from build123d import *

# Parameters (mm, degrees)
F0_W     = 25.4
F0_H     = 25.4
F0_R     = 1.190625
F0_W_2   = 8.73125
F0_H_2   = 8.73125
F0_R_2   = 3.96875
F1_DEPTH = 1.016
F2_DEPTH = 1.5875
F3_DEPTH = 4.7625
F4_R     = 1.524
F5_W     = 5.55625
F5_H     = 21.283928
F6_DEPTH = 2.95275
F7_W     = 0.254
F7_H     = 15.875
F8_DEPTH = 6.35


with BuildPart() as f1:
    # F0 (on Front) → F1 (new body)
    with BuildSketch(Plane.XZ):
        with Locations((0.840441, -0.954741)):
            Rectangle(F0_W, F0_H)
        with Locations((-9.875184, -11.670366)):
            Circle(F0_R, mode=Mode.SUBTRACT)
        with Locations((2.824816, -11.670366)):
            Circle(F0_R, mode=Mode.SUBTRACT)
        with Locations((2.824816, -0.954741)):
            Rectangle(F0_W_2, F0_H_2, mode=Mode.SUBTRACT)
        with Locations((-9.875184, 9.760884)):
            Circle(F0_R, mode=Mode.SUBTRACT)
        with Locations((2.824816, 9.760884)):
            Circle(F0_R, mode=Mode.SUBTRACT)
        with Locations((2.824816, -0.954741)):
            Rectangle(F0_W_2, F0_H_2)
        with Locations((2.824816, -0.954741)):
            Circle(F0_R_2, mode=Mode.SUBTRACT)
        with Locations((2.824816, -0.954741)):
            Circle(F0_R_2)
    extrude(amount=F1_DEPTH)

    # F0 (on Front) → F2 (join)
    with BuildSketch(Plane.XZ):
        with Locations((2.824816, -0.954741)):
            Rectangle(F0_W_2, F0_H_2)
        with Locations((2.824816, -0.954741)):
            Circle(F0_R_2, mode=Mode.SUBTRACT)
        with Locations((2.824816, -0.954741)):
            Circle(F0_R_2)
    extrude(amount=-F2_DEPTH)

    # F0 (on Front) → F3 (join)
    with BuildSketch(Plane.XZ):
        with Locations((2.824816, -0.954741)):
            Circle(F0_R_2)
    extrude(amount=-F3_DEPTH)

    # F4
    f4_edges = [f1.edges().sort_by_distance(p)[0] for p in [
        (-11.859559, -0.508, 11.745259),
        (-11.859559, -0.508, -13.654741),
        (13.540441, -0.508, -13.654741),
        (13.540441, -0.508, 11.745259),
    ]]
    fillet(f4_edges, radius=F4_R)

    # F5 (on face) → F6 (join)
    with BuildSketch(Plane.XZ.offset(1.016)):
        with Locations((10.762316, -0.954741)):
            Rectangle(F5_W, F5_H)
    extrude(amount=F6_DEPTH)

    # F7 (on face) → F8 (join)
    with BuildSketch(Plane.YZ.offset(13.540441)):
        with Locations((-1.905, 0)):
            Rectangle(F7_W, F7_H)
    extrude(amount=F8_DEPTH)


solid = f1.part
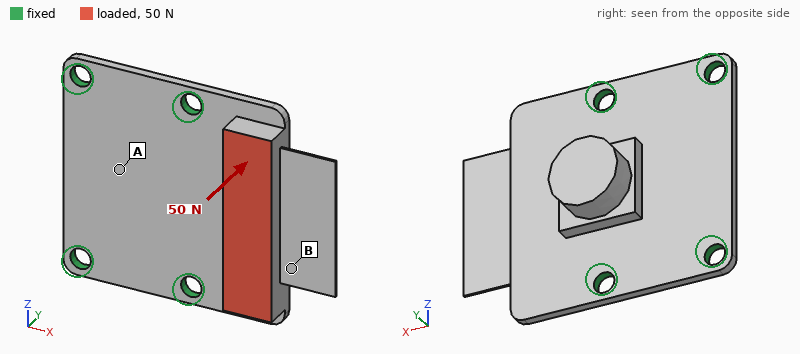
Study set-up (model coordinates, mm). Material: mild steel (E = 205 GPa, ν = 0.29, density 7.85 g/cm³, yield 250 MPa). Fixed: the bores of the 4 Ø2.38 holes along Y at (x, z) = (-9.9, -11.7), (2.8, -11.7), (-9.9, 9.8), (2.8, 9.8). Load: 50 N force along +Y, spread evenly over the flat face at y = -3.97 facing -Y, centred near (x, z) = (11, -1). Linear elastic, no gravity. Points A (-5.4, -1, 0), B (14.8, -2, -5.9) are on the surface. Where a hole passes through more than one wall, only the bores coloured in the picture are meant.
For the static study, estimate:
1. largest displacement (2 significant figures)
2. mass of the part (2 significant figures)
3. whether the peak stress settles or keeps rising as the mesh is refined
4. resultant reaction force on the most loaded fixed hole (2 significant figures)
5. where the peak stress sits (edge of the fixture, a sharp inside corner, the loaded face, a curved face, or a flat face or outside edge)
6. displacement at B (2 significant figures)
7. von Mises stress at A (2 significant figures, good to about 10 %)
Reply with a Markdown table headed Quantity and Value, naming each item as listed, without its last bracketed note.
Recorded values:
| Quantity | Value |
|---|---|
| largest displacement | 30 µm |
| mass of the part | 10 g |
| whether the peak stress settles or keeps rising as the mesh is refined | keeps rising |
| resultant reaction force on the most loaded fixed hole | 33 N |
| where the peak stress sits | edge of the fixture |
| displacement at B | 20 µm |
| von Mises stress at A | 13 MPa |
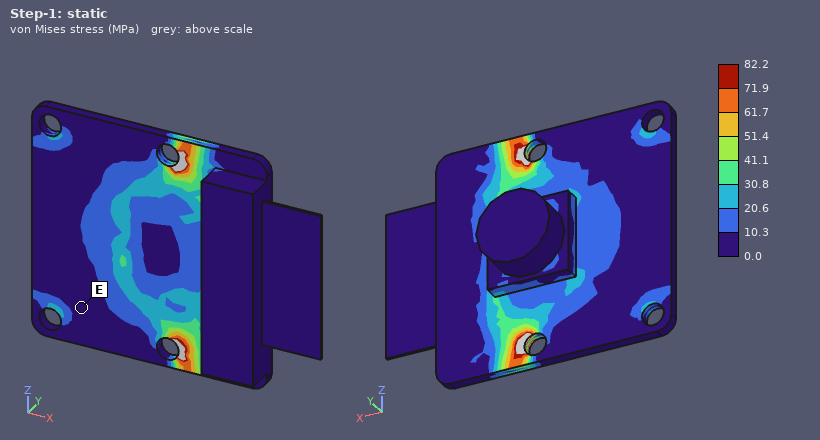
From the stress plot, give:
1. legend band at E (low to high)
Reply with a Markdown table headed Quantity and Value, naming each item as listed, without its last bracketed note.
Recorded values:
| Quantity | Value |
|---|---|
| legend band at E | 0.0 to 10.3 MPa |
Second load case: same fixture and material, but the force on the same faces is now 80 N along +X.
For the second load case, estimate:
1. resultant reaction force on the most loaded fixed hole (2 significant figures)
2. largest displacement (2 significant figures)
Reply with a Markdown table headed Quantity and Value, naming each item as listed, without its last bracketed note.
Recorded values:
| Quantity | Value |
|---|---|
| resultant reaction force on the most loaded fixed hole | 36 N |
| largest displacement | 31 µm |
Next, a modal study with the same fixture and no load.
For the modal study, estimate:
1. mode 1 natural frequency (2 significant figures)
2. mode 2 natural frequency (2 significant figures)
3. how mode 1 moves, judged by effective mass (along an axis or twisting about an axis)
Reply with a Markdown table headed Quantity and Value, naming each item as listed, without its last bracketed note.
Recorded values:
| Quantity | Value |
|---|---|
| mode 1 natural frequency | 4000 Hz |
| mode 2 natural frequency | 6000 Hz |
| how mode 1 moves, judged by effective mass | along Y |
